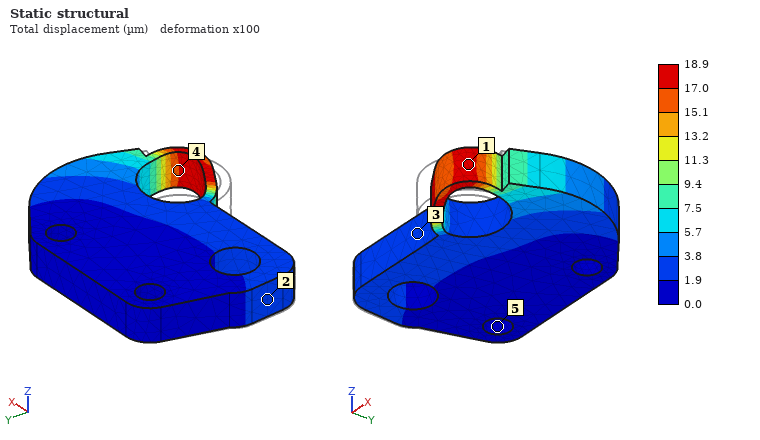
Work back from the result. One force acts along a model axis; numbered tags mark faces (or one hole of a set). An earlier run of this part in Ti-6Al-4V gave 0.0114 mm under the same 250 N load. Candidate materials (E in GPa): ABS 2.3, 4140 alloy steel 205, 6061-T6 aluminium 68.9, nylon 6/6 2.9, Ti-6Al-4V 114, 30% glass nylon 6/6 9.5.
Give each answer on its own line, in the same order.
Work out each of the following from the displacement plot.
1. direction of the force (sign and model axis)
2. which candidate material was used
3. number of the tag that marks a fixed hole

+X
6061-T6 aluminium
5
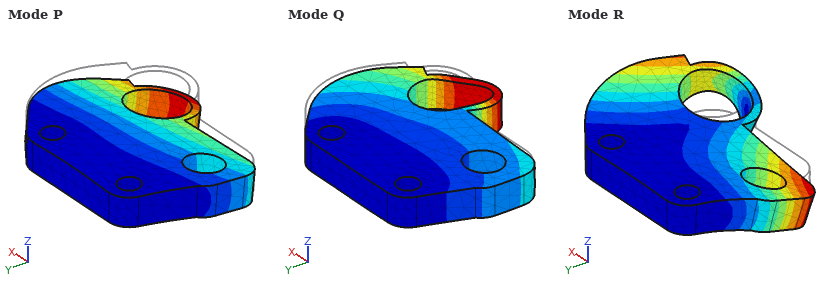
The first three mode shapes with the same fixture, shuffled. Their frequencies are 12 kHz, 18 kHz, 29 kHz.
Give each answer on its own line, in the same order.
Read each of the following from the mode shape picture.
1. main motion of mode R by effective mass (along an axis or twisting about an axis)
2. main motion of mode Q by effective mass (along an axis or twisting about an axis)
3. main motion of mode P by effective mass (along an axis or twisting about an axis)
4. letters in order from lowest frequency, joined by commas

twisting about Y
along X
along Z
P, R, Q
